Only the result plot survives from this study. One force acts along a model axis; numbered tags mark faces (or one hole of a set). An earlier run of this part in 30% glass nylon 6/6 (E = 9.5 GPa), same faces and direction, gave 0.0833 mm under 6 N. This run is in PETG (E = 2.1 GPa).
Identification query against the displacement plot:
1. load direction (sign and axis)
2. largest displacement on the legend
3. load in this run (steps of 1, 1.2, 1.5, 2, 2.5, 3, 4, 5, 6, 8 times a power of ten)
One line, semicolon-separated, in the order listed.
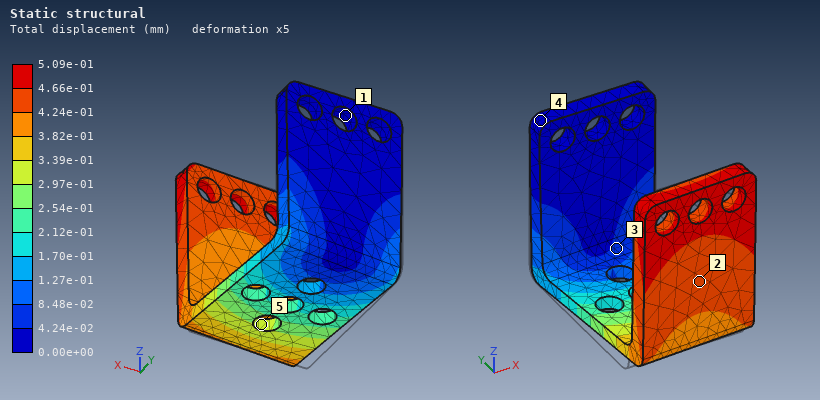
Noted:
+X; 5.09e-01 mm; 8 N
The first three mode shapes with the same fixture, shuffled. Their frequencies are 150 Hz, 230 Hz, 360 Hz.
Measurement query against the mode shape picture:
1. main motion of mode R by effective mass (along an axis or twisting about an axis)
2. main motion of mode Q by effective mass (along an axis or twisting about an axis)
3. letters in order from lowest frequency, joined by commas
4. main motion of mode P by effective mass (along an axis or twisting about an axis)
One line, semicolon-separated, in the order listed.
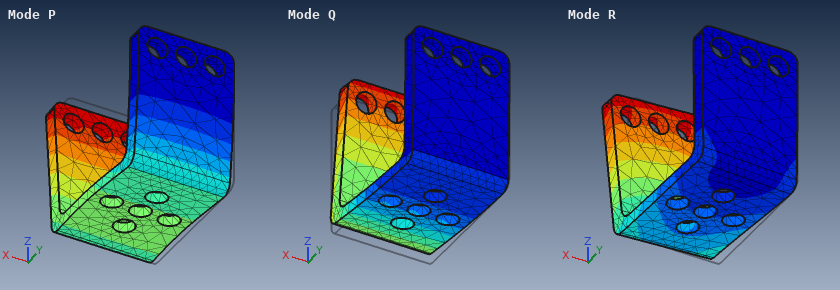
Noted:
along X; along Z; Q, R, P; along Y
